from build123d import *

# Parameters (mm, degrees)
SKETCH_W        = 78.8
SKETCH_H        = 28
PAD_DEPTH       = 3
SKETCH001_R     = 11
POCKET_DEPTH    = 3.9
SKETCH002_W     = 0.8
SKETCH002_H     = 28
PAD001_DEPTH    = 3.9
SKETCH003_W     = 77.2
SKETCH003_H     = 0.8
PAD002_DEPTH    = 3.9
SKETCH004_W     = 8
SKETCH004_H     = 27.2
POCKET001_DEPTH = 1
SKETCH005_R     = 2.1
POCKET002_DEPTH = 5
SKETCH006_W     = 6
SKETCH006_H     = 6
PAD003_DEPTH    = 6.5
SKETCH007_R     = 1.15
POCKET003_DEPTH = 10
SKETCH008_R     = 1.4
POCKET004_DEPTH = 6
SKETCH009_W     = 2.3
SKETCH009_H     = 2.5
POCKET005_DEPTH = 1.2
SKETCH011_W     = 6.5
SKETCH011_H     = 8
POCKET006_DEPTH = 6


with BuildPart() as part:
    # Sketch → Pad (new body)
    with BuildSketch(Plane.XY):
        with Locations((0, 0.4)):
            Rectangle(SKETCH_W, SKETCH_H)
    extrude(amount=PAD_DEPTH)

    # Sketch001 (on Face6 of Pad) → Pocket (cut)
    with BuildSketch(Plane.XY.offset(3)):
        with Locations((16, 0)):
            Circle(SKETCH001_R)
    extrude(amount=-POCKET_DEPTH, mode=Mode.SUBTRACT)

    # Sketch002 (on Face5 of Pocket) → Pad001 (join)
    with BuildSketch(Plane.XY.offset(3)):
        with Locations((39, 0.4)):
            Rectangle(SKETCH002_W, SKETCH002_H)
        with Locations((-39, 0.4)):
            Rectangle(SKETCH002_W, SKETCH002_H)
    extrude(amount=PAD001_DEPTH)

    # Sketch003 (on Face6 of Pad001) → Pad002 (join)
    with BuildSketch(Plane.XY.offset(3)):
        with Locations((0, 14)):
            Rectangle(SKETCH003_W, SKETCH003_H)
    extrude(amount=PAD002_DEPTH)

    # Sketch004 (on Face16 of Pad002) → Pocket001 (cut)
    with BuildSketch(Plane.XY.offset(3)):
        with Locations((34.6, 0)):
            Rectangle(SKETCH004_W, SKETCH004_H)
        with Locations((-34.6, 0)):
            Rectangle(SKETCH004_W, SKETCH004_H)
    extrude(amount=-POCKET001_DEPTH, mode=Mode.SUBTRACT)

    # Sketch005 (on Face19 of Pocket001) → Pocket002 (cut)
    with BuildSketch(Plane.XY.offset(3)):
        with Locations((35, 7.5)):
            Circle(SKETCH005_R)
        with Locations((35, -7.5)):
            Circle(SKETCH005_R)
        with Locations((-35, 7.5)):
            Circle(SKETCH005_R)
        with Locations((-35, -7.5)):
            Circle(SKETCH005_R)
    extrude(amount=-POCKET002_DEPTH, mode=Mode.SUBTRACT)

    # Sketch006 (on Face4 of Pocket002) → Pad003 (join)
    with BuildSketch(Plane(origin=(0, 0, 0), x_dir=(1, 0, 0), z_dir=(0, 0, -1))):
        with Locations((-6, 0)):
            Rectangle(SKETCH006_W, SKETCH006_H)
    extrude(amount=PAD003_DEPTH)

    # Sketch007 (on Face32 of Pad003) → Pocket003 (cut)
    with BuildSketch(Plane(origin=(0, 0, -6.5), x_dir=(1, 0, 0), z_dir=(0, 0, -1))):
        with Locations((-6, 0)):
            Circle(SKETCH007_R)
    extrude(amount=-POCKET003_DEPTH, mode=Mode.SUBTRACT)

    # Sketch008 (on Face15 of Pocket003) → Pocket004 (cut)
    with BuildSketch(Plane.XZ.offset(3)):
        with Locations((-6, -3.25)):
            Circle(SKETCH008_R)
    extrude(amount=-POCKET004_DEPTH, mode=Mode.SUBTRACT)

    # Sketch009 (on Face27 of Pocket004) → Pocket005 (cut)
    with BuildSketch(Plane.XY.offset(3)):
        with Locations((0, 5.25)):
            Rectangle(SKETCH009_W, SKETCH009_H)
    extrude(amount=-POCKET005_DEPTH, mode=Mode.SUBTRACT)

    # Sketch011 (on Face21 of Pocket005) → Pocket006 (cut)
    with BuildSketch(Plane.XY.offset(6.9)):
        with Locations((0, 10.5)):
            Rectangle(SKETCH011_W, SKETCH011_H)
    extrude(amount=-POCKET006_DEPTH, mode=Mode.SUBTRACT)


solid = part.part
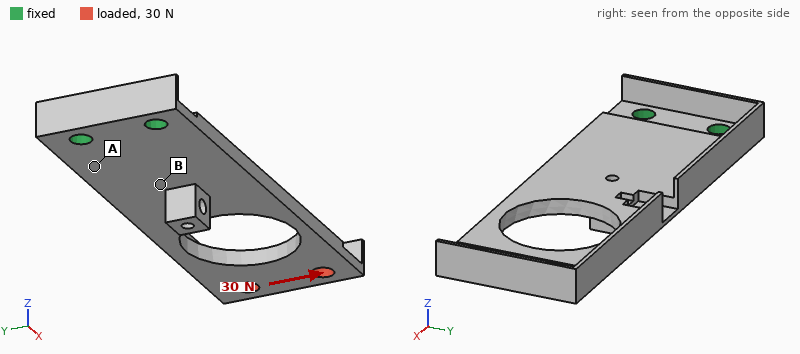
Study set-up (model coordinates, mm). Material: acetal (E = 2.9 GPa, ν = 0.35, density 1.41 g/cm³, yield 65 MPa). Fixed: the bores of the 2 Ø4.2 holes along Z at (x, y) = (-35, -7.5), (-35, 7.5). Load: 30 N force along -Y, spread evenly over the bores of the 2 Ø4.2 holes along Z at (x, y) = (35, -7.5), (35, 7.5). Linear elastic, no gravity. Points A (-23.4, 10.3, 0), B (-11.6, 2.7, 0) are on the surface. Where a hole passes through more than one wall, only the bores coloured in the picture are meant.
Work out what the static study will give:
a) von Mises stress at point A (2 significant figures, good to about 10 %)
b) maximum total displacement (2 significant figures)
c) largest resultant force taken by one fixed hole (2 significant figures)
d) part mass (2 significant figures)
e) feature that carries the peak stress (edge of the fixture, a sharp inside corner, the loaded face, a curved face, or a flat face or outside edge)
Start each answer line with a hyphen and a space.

- 4.2 MPa
- 0.79 mm
- 120 N
- 7.6 g
- a flat face or outside edge
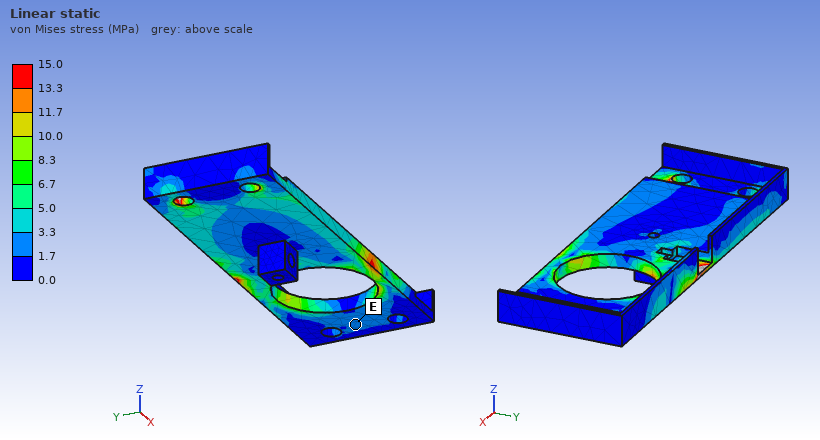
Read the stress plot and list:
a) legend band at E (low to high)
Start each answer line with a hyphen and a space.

- 1.7 to 3.3 MPa
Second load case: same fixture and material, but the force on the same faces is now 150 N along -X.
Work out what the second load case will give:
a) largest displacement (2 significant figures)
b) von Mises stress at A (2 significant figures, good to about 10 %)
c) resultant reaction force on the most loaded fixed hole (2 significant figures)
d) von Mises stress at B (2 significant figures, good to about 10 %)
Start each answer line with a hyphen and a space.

- 0.90 mm
- 3.1 MPa
- 76 N
- 2.6 MPa
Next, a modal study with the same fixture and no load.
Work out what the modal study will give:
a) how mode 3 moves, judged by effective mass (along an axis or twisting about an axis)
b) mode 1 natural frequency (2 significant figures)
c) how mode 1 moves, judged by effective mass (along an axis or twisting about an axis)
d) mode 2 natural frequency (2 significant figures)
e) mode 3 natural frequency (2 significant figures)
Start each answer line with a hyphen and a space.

- along Z
- 140 Hz
- along Z
- 550 Hz
- 630 Hz
